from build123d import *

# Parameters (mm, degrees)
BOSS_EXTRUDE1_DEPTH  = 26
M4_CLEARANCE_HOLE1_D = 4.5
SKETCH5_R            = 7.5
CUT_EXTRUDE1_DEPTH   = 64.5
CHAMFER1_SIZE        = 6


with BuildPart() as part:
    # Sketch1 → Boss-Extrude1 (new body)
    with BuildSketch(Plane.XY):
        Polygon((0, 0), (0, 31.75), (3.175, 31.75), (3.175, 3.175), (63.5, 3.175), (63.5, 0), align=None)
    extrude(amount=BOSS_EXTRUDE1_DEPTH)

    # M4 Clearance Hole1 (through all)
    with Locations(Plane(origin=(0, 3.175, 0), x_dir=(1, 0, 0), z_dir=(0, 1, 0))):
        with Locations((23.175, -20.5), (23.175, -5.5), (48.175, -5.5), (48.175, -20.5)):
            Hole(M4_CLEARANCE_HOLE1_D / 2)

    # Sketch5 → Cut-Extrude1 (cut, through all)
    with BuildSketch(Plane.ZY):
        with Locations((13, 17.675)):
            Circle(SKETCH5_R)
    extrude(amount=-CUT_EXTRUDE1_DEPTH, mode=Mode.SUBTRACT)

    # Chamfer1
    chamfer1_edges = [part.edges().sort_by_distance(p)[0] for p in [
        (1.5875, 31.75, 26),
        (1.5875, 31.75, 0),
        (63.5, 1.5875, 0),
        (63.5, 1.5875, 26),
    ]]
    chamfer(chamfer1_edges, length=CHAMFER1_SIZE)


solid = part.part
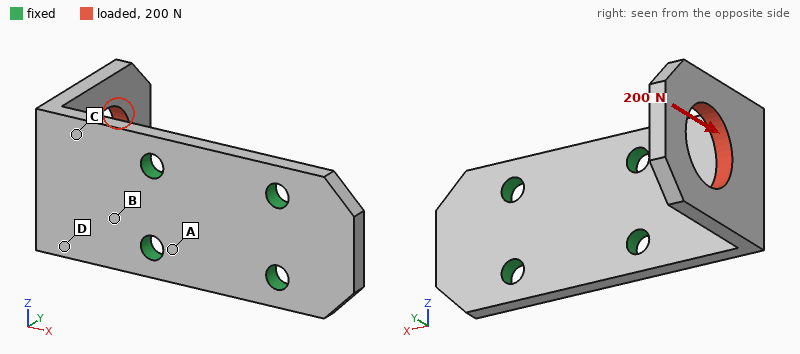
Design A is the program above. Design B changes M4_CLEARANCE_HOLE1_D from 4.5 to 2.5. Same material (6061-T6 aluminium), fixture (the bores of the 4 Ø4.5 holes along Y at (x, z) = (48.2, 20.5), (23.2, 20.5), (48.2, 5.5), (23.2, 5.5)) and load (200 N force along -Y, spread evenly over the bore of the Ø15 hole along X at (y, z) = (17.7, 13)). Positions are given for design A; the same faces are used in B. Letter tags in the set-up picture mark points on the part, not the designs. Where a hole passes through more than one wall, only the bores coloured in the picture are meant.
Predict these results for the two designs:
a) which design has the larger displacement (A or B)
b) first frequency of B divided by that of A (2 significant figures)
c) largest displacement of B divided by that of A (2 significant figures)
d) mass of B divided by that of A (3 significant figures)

B
0.95
1.2
1.02
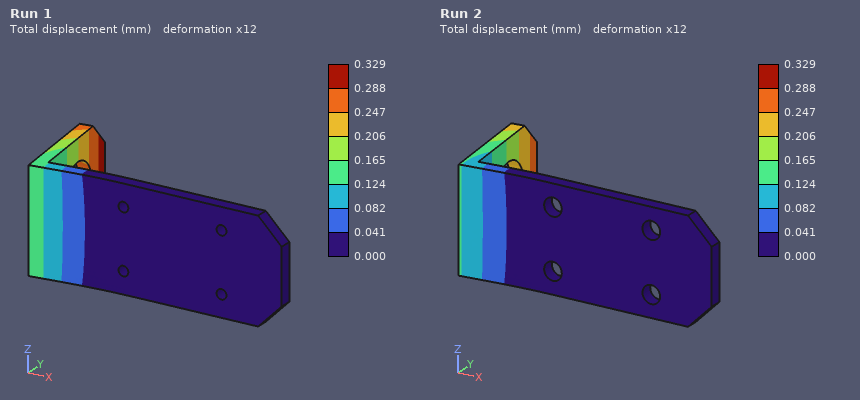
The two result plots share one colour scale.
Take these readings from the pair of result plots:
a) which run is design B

Run 1
